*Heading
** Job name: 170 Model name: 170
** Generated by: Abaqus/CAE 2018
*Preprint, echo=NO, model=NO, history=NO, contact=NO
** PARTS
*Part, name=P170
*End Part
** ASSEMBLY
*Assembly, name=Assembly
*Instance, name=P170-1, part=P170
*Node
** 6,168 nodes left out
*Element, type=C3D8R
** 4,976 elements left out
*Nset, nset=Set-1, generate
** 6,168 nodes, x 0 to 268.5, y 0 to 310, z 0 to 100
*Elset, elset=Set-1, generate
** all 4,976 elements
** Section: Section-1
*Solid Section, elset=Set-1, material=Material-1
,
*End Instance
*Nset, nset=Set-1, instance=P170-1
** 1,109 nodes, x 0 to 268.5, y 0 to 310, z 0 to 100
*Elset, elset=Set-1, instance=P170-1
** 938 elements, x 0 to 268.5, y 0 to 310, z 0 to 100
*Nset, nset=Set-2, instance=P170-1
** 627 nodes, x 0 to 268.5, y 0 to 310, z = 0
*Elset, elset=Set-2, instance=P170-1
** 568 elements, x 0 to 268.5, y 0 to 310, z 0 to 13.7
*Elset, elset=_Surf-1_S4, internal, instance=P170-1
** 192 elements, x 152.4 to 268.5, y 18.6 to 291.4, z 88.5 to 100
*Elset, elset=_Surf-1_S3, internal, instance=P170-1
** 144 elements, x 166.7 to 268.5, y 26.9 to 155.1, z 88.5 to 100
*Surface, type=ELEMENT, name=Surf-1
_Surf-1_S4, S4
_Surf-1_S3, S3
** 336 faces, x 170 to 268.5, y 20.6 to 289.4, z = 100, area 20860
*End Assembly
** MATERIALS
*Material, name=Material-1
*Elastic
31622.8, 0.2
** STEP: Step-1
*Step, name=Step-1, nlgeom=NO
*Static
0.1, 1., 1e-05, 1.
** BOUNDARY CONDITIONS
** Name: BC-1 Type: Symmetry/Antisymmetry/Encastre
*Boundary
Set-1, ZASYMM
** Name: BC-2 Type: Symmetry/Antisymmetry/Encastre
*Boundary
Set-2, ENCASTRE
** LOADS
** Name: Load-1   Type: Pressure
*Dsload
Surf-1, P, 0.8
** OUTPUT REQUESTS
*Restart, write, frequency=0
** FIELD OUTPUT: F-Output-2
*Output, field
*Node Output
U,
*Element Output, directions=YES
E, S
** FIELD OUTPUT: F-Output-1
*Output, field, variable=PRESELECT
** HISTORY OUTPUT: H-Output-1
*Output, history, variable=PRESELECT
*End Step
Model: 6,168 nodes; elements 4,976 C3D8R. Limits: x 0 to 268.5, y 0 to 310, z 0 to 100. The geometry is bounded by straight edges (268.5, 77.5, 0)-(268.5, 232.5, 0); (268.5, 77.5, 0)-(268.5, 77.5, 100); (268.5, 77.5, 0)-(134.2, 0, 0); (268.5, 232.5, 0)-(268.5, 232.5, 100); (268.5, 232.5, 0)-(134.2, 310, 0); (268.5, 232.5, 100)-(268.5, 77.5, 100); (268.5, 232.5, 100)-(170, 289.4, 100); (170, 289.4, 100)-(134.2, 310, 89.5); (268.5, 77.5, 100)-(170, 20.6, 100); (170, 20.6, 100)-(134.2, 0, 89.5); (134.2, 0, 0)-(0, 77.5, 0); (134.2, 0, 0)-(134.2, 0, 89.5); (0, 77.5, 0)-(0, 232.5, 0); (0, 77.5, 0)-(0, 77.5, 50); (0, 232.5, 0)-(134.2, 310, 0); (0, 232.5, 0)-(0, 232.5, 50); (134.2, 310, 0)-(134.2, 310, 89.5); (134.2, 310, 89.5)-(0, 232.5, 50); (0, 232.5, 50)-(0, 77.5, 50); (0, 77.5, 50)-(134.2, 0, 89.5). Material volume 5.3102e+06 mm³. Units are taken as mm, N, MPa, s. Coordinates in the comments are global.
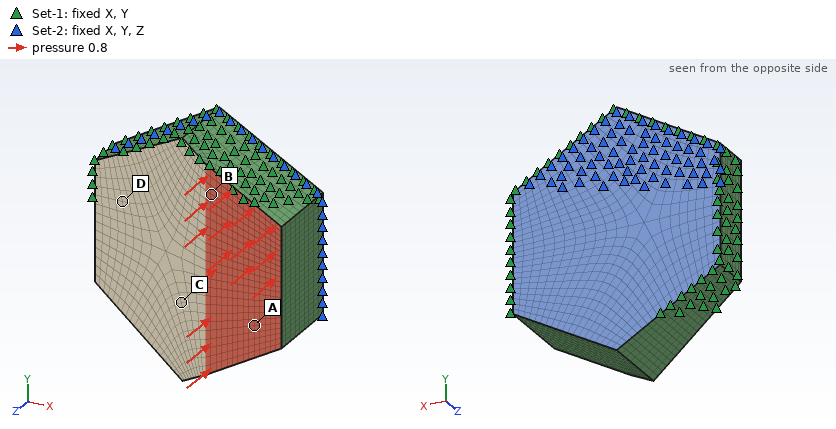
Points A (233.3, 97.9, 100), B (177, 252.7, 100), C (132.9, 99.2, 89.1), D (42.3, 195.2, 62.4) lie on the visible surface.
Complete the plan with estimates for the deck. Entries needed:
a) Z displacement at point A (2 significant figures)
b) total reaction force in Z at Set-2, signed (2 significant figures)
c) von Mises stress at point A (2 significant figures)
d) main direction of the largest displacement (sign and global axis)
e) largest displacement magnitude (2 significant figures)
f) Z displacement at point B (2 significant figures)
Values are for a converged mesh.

-0.0022 mm
17000 N
0.52 MPa
-Z
0.0023 mm
-0.0014 mm
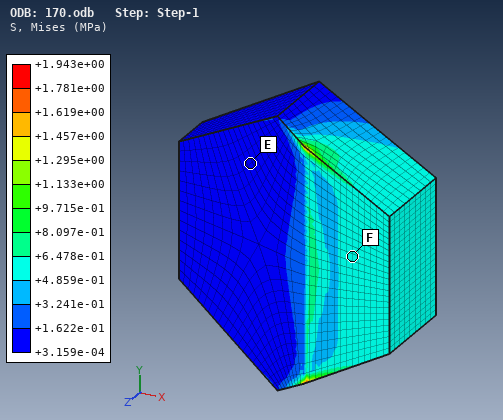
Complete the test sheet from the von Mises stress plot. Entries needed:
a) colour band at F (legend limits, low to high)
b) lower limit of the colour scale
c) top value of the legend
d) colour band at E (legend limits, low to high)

+4.859e-01 to +6.478e-01 MPa
+3.159e-04 MPa
+1.943e+00 MPa
+3.159e-04 to +1.622e-01 MPa
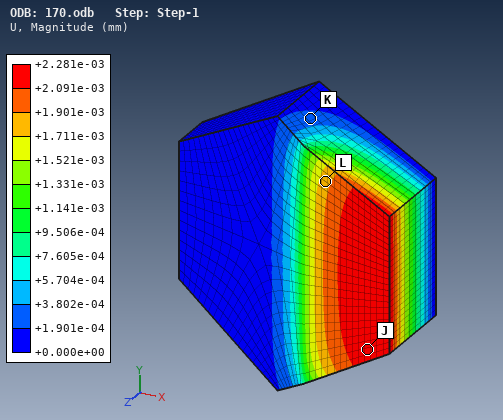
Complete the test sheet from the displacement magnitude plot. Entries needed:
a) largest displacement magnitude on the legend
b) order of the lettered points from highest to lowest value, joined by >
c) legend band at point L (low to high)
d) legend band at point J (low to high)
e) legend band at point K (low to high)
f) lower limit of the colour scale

+2.281e-03 mm
J > L > K
+1.711e-03 to +1.901e-03 mm
+2.091e-03 to +2.281e-03 mm
+1.901e-04 to +3.802e-04 mm
+0.000e+00 mm
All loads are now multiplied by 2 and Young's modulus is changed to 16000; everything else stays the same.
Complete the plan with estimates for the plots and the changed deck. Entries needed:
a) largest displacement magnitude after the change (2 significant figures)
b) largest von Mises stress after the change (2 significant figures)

0.0090 mm
3.9 MPa
